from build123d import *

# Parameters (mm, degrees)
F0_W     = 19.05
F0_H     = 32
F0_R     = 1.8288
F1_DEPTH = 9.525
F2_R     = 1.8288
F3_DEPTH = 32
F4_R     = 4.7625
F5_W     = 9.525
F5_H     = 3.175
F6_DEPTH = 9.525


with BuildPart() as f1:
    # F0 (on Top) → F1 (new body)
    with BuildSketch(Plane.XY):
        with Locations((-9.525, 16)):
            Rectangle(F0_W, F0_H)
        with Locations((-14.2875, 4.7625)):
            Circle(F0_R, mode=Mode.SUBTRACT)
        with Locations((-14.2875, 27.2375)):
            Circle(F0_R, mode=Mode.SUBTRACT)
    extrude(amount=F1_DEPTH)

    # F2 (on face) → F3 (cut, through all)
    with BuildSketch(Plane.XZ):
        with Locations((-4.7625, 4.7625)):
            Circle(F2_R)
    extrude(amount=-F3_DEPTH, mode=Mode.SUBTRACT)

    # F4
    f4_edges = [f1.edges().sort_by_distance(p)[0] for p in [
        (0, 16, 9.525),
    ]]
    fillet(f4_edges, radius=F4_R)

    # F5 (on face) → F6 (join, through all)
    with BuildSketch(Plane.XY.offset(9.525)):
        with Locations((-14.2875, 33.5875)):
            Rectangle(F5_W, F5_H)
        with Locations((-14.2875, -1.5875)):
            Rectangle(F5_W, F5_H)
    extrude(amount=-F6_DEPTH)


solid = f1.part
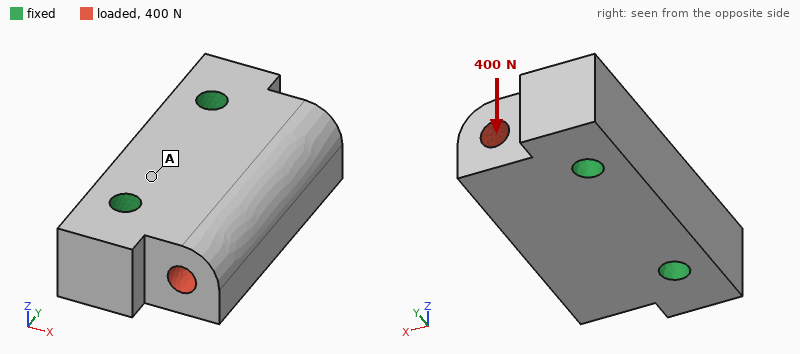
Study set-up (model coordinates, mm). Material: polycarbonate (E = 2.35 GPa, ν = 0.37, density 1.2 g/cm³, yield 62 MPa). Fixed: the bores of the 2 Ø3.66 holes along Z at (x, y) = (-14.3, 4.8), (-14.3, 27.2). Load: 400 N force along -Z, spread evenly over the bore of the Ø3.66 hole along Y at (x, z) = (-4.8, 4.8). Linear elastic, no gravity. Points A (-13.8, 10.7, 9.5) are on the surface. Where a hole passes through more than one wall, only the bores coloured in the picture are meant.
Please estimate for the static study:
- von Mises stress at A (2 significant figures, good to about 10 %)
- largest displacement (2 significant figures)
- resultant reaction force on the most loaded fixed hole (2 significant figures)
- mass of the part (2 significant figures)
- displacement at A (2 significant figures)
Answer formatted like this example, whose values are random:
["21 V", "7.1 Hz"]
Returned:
["3.0 MPa", "90 µm", "200 N", "6.8 g", "18 µm"]
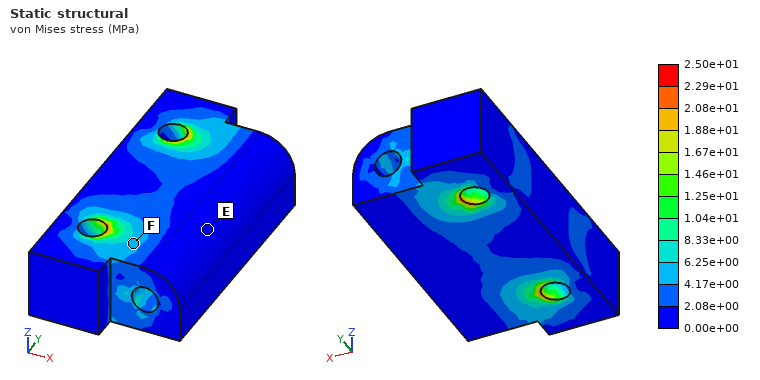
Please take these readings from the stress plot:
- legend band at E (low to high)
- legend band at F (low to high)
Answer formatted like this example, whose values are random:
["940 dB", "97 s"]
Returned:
["0.00e+00 to 2.08e+00 MPa", "4.17e+00 to 6.25e+00 MPa"]
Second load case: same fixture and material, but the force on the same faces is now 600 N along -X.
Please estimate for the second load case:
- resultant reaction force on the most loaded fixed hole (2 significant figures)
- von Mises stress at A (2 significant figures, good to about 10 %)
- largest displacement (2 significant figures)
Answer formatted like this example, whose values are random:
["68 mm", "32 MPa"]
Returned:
["310 N", "1.5 MPa", "20 µm"]
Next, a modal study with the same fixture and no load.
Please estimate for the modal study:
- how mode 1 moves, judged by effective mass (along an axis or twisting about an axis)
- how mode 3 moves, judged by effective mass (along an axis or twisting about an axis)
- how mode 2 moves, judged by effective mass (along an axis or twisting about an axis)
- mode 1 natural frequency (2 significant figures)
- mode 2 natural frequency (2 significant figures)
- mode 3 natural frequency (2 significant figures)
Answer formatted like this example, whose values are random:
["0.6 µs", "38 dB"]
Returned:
["along Z", "along Y", "twisting about X", "7400 Hz", "11 kHz", "13 kHz"]
